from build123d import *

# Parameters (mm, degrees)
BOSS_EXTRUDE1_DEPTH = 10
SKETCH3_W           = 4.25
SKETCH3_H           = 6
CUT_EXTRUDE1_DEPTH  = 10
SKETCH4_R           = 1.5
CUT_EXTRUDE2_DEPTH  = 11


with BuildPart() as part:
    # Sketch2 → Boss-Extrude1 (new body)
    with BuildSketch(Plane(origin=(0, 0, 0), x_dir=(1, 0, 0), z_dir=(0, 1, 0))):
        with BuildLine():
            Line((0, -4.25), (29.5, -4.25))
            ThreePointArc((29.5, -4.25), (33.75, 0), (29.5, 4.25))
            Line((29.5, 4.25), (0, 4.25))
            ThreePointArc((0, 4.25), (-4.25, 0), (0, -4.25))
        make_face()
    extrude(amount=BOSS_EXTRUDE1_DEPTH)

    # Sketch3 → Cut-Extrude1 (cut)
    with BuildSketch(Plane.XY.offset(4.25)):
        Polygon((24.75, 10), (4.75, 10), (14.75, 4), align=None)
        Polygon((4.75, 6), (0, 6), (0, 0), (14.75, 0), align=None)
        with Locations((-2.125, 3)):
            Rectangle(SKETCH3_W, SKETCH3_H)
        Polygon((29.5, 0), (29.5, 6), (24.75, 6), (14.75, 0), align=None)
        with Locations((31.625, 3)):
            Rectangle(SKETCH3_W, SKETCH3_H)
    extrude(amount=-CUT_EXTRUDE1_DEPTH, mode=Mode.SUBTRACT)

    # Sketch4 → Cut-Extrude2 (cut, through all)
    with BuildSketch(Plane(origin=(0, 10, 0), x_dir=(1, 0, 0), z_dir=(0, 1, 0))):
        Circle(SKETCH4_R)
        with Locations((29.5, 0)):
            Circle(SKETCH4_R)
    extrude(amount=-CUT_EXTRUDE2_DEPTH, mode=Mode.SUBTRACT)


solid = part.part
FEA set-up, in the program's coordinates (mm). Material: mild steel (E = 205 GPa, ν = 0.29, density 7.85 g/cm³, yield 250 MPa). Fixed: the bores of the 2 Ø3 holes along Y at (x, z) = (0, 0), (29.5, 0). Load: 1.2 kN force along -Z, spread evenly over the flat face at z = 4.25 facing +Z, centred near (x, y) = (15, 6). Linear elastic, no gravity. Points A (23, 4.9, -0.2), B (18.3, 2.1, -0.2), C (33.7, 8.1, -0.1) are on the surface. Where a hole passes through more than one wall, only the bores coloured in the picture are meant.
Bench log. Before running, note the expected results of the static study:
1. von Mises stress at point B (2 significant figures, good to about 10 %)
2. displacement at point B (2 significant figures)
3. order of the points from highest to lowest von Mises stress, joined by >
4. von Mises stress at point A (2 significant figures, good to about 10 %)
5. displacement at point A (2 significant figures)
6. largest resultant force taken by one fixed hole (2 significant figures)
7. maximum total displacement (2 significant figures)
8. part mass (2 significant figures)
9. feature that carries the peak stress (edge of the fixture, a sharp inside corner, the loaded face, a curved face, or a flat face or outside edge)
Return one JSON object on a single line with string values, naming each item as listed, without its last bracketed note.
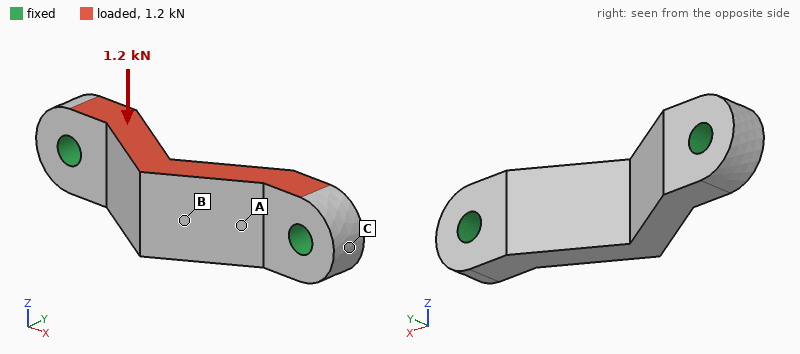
{"von Mises stress at point B": "38 MPa", "displacement at point B": "11 µm", "order of the points from highest to lowest von Mises stress, joined by >": "A > B > C", "von Mises stress at point A": "67 MPa", "displacement at point A": "5.6 µm", "largest resultant force taken by one fixed hole": "600 N", "maximum total displacement": "15 µm", "part mass": "9.2 g", "feature that carries the peak stress": "edge of the fixture"}
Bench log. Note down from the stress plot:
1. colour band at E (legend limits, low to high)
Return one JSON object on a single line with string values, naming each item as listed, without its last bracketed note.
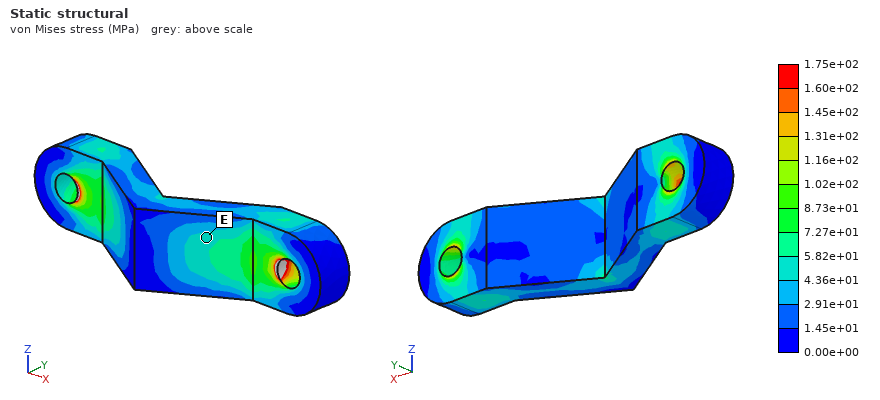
{"colour band at E": "4.36e+01 to 5.82e+01 MPa"}
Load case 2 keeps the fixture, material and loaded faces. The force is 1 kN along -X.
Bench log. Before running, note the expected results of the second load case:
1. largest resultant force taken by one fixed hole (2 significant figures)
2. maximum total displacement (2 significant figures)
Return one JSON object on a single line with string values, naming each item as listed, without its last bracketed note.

{"largest resultant force taken by one fixed hole": "520 N", "maximum total displacement": "1.9 µm"}
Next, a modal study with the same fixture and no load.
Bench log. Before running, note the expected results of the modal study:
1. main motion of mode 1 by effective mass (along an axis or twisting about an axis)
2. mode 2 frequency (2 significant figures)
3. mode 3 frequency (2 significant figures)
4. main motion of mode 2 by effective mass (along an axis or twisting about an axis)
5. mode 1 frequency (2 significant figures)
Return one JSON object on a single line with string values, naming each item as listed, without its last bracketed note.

{"main motion of mode 1 by effective mass": "along Z", "mode 2 frequency": "32 kHz", "mode 3 frequency": "48 kHz", "main motion of mode 2 by effective mass": "along Y", "mode 1 frequency": "21 kHz"}
